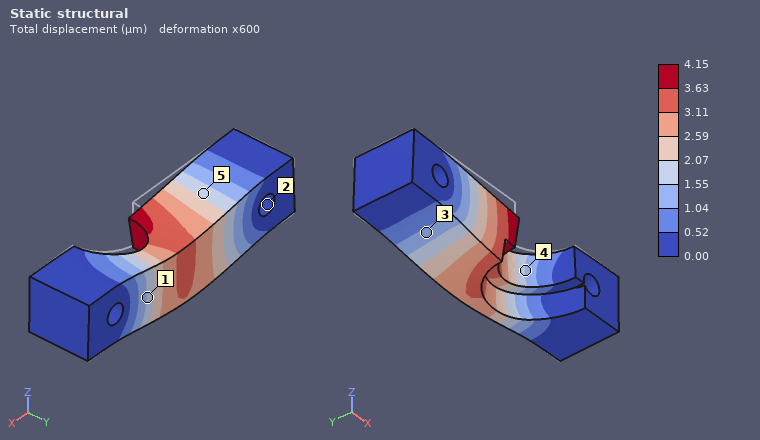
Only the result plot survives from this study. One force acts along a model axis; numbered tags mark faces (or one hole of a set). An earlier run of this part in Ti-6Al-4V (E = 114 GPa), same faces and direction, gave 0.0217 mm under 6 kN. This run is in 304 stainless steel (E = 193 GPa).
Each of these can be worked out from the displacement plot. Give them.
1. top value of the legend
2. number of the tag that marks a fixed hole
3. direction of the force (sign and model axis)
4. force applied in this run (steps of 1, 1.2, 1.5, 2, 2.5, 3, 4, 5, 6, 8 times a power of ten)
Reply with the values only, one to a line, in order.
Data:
4.15 µm
2
-Z
2 kN
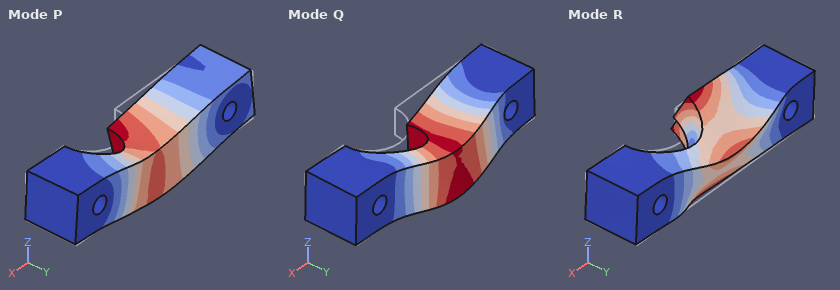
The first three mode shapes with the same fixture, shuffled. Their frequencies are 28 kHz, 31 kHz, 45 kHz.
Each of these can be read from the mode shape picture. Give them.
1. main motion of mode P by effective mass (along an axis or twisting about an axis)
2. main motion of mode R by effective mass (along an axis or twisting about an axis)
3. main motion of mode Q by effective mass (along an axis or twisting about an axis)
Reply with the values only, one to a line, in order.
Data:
along Z
twisting about X
along Y
